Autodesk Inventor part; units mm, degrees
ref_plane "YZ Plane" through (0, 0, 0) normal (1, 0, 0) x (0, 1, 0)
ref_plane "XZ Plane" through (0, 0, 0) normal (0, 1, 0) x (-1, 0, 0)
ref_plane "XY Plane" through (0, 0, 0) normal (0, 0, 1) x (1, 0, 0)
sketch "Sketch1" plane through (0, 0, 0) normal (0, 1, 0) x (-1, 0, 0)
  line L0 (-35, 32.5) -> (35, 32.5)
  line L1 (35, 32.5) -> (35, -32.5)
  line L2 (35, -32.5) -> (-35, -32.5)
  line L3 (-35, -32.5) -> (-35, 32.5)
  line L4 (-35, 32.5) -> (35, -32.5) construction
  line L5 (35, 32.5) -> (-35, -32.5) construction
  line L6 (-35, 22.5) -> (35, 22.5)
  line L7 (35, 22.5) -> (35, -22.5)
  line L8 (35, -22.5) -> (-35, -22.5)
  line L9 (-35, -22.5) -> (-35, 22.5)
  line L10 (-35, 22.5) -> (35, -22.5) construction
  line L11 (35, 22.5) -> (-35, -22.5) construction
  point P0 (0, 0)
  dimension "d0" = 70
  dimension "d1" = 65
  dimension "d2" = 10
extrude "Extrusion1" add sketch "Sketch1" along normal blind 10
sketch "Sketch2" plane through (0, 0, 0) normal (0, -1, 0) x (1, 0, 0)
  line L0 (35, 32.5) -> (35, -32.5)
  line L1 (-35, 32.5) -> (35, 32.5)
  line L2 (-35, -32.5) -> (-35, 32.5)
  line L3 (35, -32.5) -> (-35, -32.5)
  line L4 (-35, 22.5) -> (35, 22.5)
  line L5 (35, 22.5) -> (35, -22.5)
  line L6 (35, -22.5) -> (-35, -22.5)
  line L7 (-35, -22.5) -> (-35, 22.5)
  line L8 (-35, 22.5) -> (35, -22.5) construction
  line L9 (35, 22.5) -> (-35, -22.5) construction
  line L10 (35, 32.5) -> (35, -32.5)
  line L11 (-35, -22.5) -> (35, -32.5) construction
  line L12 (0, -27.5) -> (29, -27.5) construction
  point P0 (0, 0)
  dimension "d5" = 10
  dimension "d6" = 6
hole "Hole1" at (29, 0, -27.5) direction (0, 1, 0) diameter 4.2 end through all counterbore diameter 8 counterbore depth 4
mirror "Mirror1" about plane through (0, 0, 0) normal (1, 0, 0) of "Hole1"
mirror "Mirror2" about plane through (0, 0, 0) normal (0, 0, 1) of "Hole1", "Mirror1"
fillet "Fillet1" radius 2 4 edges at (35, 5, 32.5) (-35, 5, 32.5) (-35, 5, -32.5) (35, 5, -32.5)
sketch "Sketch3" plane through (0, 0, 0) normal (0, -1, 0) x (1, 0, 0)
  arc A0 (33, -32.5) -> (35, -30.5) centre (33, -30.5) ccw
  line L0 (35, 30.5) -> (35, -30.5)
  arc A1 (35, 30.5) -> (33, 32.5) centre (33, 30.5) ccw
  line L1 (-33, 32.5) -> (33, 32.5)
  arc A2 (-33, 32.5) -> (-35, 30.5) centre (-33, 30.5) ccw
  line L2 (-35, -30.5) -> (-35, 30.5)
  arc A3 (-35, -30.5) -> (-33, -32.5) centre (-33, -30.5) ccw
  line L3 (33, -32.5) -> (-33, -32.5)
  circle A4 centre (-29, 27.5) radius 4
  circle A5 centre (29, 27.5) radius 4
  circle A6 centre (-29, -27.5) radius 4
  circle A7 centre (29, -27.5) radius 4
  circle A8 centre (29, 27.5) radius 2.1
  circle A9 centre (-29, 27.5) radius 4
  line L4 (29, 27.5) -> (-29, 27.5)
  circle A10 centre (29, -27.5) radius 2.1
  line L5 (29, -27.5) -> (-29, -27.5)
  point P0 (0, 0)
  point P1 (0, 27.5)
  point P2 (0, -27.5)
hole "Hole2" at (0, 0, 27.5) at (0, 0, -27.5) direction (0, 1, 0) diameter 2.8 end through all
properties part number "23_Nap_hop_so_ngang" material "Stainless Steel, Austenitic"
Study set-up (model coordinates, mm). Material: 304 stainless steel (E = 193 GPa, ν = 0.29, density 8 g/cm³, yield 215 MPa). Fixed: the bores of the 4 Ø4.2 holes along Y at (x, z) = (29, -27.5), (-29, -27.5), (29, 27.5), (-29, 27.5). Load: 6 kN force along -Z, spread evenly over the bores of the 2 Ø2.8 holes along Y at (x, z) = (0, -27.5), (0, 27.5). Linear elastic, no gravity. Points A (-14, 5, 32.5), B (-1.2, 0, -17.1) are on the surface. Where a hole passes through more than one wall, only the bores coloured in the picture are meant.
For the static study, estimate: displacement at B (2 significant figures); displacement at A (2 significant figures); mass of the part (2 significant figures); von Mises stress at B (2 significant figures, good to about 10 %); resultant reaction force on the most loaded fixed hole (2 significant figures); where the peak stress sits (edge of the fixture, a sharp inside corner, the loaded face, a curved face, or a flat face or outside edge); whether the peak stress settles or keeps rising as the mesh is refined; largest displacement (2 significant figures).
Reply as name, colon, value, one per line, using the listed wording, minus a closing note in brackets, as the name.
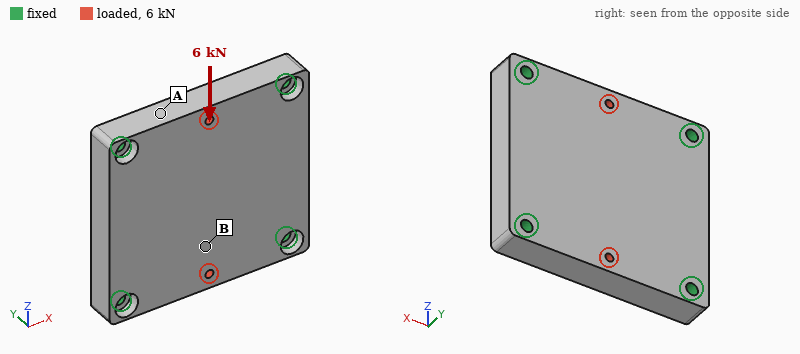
displacement at B: 2.7 µm
displacement at A: 2.1 µm
mass of the part: 350 g
von Mises stress at B: 14 MPa
resultant reaction force on the most loaded fixed hole: 1.6 kN
where the peak stress sits: edge of the fixture
whether the peak stress settles or keeps rising as the mesh is refined: keeps rising
largest displacement: 4.3 µm
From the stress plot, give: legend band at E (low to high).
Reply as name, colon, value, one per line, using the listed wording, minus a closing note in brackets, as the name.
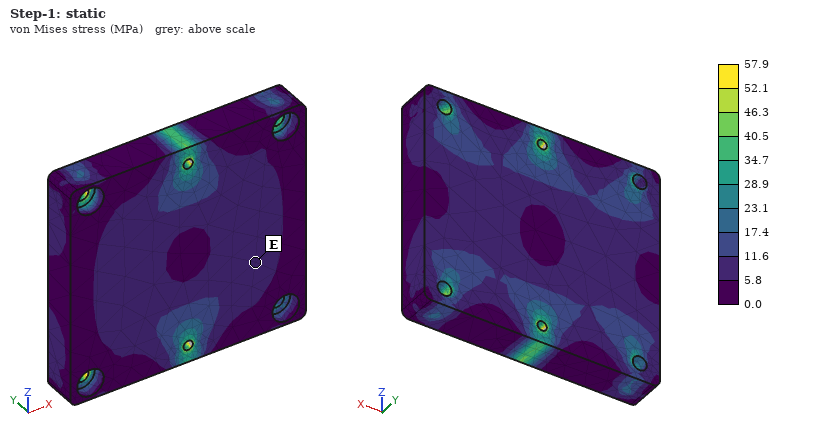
legend band at E: 5.8 to 11.6 MPa
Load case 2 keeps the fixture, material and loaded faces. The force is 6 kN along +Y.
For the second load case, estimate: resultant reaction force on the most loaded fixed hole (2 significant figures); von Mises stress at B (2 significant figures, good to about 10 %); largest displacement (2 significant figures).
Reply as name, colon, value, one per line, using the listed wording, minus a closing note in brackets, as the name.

resultant reaction force on the most loaded fixed hole: 1.9 kN
von Mises stress at B: 54 MPa
largest displacement: 22 µm
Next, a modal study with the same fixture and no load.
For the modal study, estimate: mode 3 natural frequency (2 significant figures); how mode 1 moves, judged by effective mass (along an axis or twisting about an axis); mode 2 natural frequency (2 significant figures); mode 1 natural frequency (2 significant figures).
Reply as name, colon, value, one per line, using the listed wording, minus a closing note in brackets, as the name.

mode 3 natural frequency: 13 kHz
how mode 1 moves, judged by effective mass: along Y
mode 2 natural frequency: 12 kHz
mode 1 natural frequency: 7400 Hz
